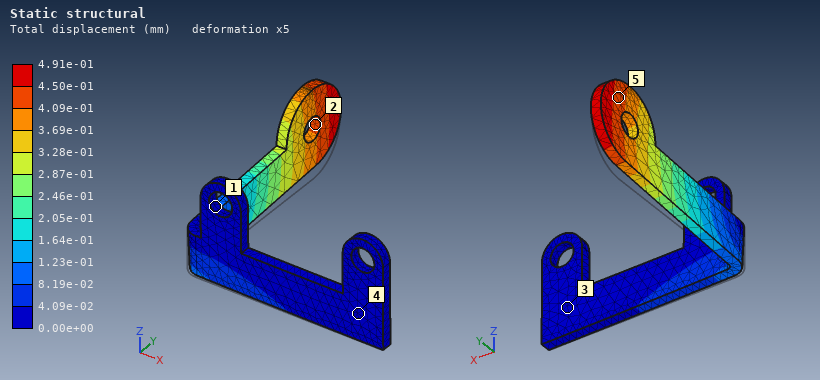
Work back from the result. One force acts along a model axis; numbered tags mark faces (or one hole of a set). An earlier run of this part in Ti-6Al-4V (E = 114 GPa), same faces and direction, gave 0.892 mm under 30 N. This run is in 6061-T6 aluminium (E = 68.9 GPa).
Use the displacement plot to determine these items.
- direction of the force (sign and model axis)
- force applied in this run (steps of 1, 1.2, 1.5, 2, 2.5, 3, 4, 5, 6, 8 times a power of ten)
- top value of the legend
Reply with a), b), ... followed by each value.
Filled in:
a) +Z
b) 10 N
c) 4.91e-01 mm
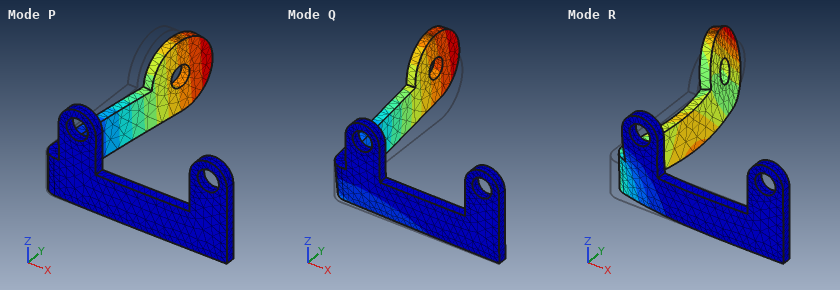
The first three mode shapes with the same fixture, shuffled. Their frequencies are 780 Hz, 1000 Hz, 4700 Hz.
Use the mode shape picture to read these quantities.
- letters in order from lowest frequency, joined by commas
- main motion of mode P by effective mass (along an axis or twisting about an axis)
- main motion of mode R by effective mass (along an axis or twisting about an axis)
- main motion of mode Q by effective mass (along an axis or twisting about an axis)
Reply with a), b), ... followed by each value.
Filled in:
a) P, Q, R
b) along X
c) along Y
d) along Z
